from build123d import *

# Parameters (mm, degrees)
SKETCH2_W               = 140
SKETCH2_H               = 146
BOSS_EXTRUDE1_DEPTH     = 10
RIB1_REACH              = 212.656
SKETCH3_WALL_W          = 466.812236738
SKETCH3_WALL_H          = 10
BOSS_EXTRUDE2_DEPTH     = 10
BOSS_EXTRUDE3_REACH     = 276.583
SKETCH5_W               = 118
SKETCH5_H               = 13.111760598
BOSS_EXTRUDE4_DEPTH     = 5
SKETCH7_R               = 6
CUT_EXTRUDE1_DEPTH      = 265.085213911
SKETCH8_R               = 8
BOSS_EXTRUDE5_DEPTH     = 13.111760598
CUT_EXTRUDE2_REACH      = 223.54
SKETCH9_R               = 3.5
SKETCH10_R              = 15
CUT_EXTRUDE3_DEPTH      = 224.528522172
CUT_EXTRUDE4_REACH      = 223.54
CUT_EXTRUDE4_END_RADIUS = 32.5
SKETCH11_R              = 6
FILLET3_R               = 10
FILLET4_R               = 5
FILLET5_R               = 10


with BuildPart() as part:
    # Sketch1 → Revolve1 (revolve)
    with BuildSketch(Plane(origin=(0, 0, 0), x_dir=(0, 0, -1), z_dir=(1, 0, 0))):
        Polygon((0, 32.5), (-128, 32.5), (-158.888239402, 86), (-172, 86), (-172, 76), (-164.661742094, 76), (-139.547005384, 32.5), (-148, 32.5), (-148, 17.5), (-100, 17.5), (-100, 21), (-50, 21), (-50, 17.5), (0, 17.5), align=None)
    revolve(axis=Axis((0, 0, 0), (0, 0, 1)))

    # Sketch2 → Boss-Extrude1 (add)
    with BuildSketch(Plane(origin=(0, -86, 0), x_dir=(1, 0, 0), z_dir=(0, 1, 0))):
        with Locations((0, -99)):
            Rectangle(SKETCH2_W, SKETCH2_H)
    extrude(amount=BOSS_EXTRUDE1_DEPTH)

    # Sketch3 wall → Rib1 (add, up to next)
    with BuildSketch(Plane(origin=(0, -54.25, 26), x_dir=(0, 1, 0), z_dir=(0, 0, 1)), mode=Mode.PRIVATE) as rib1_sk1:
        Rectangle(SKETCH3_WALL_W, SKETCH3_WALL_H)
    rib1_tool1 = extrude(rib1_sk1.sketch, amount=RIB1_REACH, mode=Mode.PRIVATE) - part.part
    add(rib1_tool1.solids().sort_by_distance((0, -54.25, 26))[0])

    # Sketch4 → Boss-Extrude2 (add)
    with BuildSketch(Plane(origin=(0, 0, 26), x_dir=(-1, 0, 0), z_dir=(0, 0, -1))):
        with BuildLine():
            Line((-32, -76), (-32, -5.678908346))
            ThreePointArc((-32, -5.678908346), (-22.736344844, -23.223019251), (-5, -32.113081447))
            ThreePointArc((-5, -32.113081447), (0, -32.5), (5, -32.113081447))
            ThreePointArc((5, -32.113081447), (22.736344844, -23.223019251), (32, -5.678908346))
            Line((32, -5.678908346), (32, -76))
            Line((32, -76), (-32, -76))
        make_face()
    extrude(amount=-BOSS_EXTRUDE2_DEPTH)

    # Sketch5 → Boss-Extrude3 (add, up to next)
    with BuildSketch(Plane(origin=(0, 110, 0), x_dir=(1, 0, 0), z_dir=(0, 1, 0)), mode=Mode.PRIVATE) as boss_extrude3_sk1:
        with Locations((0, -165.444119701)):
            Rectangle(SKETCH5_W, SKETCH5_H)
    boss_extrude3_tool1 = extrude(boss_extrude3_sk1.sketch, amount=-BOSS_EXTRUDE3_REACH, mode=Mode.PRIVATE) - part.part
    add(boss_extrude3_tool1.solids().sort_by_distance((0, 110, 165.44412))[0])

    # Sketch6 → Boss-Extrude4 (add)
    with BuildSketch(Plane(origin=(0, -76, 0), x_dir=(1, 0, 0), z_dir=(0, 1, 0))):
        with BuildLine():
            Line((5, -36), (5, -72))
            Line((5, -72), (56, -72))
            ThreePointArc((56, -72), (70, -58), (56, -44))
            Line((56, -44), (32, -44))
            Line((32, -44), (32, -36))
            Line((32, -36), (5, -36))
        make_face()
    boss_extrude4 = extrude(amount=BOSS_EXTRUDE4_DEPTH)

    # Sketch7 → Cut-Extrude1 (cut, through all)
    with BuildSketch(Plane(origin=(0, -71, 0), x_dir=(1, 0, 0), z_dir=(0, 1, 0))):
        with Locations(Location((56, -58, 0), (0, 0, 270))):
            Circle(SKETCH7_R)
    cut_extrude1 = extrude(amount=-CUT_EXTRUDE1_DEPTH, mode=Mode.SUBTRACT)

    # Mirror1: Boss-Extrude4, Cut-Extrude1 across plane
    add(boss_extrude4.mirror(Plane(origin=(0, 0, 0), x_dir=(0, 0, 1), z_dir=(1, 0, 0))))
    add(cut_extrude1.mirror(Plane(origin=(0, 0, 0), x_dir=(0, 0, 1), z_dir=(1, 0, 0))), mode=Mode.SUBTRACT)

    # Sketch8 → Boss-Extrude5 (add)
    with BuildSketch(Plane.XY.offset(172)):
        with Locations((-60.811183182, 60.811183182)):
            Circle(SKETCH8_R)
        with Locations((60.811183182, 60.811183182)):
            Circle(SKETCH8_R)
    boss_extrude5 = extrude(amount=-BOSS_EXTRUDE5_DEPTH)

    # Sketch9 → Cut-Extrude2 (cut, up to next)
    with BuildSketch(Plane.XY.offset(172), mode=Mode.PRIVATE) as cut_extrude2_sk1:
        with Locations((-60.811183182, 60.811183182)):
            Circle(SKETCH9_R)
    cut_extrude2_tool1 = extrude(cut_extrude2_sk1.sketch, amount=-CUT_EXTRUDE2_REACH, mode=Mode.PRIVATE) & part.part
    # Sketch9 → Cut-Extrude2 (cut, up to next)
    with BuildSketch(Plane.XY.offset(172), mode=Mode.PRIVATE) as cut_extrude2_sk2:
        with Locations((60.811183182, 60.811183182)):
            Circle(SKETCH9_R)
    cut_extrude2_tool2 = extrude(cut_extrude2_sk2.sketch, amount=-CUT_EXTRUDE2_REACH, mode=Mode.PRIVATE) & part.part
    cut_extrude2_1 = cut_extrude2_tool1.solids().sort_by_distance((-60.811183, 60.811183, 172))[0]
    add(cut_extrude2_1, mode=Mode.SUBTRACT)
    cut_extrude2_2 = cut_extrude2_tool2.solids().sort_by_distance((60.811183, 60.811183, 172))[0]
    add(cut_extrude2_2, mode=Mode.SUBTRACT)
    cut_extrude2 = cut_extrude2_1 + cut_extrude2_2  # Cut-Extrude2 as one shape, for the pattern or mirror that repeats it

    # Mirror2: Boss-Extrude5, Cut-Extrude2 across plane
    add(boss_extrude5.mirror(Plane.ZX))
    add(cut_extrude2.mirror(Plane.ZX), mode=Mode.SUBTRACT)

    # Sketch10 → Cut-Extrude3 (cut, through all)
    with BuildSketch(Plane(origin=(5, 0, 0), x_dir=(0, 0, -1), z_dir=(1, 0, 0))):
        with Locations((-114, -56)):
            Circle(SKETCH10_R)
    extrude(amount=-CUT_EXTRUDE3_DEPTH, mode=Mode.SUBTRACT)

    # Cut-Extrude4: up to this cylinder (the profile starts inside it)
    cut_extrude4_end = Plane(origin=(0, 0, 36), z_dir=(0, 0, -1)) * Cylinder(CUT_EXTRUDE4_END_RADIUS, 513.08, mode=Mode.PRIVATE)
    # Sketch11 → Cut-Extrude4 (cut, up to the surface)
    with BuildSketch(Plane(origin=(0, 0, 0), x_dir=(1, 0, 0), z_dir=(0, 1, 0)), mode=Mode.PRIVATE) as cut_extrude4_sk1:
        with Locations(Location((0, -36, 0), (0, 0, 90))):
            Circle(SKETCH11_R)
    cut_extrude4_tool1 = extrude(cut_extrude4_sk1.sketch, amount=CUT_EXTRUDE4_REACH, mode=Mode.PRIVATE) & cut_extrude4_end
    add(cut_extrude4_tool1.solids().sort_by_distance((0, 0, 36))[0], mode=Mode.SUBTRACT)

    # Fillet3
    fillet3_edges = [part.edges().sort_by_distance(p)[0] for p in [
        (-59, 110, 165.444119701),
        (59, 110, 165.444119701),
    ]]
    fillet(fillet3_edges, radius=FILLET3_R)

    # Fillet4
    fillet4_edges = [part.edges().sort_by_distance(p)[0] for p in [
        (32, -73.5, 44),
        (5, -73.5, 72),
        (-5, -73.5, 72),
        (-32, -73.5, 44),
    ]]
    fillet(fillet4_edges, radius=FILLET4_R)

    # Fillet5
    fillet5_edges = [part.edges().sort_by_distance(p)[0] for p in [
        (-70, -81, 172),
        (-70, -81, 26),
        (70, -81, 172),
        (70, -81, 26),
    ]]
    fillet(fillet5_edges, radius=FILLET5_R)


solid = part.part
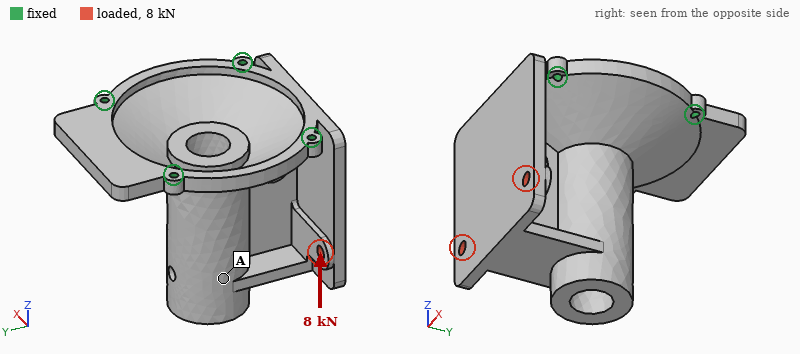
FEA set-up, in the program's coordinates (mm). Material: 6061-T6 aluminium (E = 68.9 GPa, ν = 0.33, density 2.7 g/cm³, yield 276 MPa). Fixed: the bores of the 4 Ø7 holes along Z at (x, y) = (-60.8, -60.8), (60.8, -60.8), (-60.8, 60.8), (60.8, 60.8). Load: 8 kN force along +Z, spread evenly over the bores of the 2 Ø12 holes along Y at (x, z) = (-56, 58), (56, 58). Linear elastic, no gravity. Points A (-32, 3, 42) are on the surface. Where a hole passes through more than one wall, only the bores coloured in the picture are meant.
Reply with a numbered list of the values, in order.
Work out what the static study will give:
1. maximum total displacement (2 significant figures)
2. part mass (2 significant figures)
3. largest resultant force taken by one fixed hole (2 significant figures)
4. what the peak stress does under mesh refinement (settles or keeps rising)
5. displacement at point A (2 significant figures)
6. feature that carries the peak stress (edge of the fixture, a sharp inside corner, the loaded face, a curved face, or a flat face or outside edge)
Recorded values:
1. 89 µm
2. 2.5 kg
3. 6.9 kN
4. keeps rising
5. 53 µm
6. edge of the fixture
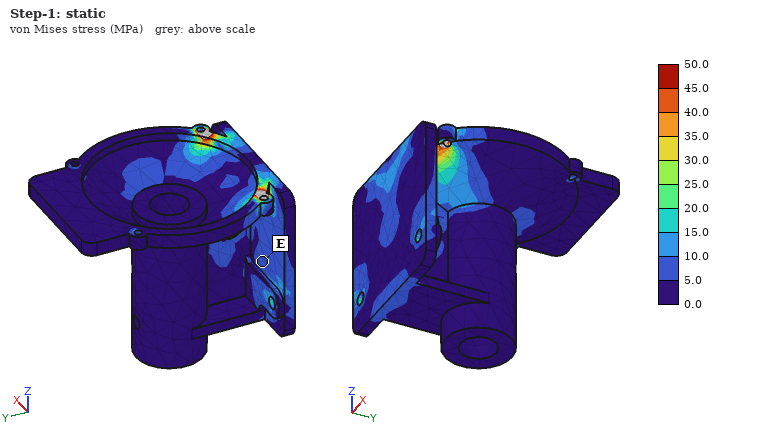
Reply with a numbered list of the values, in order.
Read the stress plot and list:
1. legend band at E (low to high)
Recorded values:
1. 5.0 to 10.0 MPa
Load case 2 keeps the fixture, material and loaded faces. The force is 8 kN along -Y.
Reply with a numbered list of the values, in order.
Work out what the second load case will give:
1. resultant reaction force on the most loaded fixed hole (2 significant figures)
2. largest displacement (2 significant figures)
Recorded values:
1. 5.6 kN
2. 0.29 mm
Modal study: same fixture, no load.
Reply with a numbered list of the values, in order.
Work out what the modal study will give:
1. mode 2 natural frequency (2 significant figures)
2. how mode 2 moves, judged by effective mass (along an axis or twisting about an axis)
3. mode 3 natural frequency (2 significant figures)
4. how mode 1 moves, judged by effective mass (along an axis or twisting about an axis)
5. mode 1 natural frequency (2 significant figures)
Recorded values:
1. 1200 Hz
2. along Y
3. 1900 Hz
4. along X
5. 1100 Hz
